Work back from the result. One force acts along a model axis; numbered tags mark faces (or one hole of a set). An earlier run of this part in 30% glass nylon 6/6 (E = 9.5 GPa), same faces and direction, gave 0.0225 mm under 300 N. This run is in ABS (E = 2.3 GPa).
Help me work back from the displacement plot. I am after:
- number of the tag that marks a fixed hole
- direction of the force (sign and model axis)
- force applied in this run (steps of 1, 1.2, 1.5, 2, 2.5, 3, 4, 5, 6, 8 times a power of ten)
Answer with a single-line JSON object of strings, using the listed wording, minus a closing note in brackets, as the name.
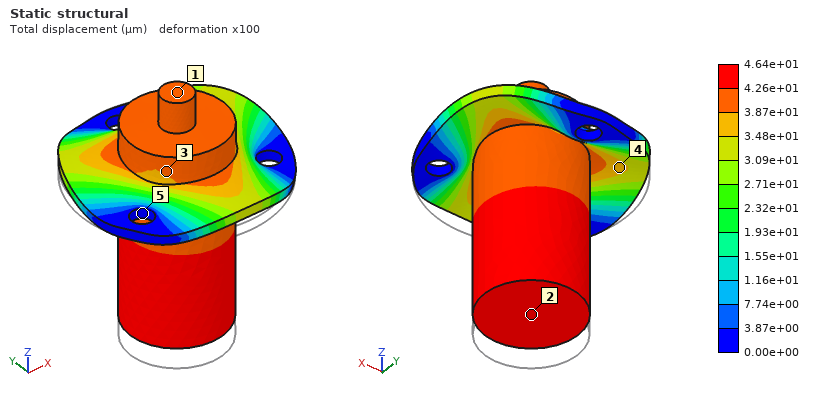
{"number of the tag that marks a fixed hole": "5", "direction of the force": "+Z", "force applied in this run": "150 N"}
